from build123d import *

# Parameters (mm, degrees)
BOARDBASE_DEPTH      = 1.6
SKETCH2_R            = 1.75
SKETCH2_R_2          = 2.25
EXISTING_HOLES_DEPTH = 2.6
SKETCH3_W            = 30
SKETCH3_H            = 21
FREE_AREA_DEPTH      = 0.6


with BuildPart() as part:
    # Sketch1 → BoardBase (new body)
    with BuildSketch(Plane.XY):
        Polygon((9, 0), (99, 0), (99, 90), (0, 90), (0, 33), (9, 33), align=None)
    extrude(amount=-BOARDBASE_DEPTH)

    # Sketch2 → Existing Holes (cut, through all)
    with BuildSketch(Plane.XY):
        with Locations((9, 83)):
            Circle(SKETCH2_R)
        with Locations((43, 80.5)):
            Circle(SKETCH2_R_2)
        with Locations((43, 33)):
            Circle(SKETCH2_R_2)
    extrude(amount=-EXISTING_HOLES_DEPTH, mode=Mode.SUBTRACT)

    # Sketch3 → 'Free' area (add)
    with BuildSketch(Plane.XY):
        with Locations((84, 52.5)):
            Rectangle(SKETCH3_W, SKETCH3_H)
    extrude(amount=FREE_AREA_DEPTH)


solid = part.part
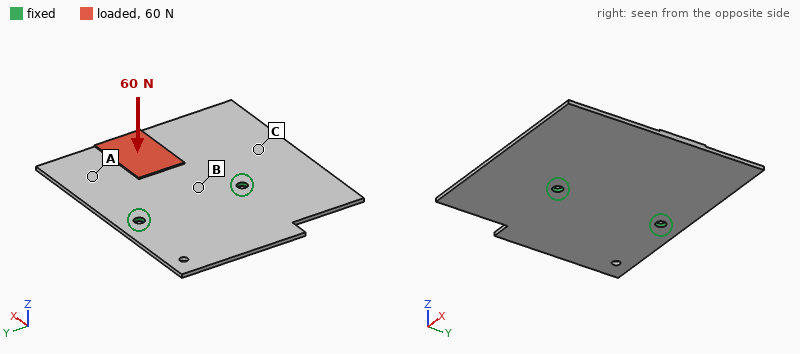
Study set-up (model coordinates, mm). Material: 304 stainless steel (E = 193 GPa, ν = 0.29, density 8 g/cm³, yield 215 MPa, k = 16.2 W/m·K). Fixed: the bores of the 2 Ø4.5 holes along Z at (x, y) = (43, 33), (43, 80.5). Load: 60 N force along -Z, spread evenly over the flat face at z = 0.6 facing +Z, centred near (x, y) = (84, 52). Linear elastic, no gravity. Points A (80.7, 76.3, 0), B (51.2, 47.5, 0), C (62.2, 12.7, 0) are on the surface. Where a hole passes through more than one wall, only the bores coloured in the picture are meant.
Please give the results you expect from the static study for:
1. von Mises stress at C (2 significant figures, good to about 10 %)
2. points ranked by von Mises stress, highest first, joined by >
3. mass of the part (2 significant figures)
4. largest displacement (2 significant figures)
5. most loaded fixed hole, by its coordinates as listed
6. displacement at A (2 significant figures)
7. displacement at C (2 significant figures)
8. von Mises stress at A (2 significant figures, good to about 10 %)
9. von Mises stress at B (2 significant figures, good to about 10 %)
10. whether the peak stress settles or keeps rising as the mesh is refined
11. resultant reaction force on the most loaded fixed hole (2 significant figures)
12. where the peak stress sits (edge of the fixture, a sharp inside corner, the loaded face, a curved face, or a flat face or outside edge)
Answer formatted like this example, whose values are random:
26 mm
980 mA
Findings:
29 MPa
B > C > A
110 g
0.44 mm
(43, 33)
0.24 mm
0.072 mm
10 MPa
47 MPa
keeps rising
34 N
edge of the fixture
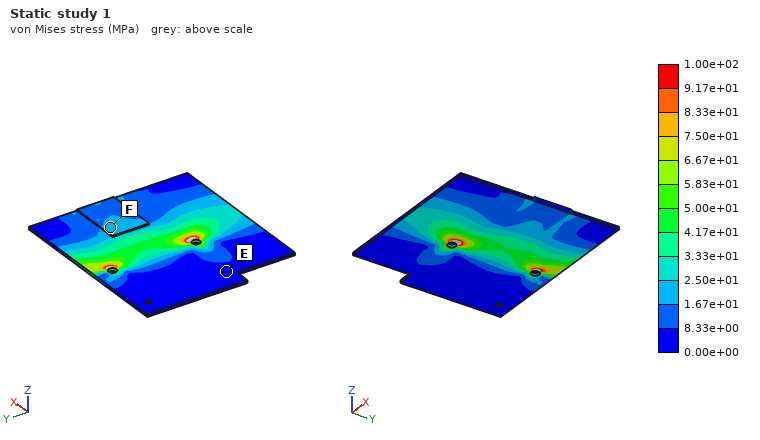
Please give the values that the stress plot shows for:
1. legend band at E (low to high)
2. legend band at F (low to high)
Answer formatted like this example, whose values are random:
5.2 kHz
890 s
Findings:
0.00e+00 to 8.33e+00 MPa
1.67e+01 to 2.50e+01 MPa
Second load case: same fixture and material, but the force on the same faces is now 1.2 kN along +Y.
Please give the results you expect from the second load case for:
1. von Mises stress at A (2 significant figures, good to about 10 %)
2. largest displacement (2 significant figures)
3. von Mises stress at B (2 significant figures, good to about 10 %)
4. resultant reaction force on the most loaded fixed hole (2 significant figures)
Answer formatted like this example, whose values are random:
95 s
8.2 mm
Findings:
28 MPa
0.16 mm
37 MPa
1.2 kN
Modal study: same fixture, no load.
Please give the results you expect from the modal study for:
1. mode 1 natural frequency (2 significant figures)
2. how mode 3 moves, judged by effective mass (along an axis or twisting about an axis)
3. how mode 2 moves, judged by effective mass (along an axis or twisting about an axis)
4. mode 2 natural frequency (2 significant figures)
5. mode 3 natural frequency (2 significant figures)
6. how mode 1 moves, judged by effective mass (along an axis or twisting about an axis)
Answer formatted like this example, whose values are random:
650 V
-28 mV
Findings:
360 Hz
along Z
twisting about X
660 Hz
720 Hz
along Z
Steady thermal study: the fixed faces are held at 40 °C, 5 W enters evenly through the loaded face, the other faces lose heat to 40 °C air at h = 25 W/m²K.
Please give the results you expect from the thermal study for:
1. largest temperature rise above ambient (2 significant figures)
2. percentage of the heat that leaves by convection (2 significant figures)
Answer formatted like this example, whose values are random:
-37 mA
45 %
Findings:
52 K
85 %
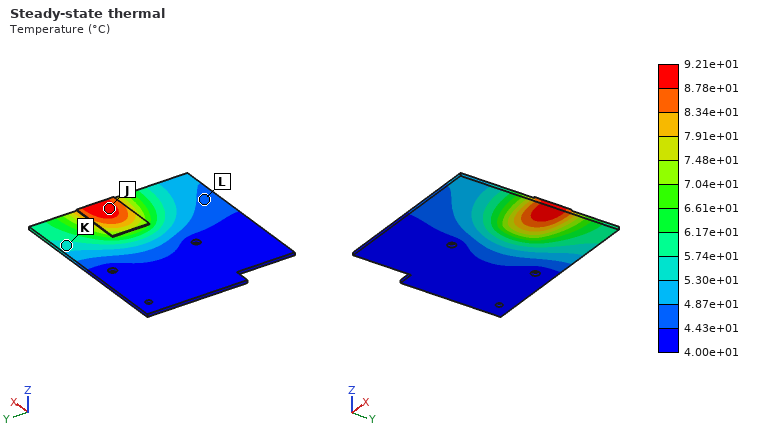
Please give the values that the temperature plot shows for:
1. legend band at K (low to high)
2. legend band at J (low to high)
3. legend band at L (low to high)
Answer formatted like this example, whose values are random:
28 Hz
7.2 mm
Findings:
5.30e+01 to 5.74e+01 °C
8.78e+01 to 9.21e+01 °C
4.43e+01 to 4.87e+01 °C
